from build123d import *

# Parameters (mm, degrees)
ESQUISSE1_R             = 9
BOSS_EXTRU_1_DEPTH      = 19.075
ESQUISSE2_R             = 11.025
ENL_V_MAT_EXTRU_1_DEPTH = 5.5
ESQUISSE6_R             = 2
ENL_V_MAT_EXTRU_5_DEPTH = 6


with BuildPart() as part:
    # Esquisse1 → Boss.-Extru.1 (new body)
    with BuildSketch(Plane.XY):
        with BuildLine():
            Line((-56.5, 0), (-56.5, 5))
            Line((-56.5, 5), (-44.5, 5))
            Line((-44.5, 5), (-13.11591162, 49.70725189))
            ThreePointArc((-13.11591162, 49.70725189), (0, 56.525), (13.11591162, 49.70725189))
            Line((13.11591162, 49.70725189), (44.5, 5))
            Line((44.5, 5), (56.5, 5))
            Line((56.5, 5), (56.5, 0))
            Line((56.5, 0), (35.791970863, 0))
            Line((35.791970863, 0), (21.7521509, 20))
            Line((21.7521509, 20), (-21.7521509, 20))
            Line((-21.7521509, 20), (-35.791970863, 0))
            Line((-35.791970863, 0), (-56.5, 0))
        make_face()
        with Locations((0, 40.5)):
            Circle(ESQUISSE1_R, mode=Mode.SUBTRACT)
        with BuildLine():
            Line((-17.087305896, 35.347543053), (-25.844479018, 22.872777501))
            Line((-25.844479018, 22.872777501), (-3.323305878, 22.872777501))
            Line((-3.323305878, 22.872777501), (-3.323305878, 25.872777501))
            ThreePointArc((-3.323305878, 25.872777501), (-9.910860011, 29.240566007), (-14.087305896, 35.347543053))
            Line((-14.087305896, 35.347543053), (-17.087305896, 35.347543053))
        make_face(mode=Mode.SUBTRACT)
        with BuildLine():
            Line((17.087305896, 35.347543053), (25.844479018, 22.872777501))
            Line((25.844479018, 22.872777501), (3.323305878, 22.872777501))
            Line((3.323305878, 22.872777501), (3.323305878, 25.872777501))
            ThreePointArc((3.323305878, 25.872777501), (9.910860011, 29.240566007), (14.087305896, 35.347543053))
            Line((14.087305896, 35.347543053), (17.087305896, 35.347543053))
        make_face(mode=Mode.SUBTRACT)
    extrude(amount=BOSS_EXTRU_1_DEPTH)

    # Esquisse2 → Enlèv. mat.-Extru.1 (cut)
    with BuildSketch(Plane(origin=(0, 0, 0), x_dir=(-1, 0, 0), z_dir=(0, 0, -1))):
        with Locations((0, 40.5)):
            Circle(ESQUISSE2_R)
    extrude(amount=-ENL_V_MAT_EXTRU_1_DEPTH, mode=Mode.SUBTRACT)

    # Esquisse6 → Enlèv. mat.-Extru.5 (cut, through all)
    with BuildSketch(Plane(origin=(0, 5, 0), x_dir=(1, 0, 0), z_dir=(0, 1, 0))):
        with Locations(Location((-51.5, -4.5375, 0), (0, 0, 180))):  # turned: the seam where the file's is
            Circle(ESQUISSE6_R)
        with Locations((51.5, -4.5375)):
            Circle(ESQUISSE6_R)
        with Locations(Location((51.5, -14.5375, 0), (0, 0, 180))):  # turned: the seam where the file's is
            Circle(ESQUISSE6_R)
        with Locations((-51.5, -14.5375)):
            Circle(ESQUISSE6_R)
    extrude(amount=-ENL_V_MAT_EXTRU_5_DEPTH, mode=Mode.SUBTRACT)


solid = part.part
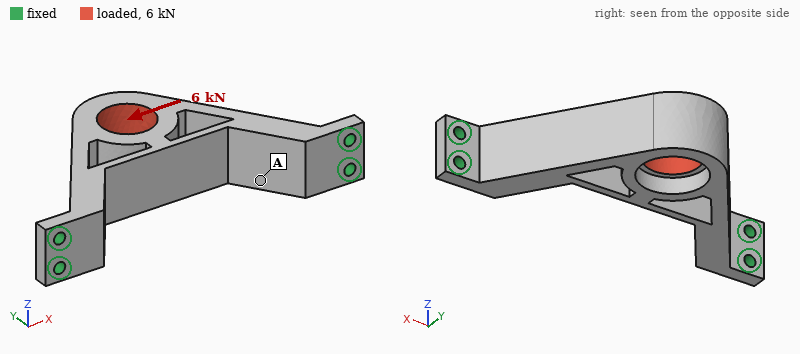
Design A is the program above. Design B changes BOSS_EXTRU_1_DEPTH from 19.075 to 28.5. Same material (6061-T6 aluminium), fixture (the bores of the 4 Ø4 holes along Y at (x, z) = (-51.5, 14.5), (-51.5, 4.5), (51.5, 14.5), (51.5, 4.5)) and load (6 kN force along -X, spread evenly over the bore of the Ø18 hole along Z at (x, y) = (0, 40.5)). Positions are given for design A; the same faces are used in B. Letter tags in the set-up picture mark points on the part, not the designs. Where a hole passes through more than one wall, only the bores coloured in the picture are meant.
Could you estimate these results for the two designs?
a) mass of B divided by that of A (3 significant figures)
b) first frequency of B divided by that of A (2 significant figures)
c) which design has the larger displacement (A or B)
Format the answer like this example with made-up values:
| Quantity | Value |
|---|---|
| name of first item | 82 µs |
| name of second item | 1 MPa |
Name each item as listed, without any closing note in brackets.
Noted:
| Quantity | Value |
|---|---|
| mass of B divided by that of A | 1.51 |
| first frequency of B divided by that of A | 0.97 |
| which design has the larger displacement | A |
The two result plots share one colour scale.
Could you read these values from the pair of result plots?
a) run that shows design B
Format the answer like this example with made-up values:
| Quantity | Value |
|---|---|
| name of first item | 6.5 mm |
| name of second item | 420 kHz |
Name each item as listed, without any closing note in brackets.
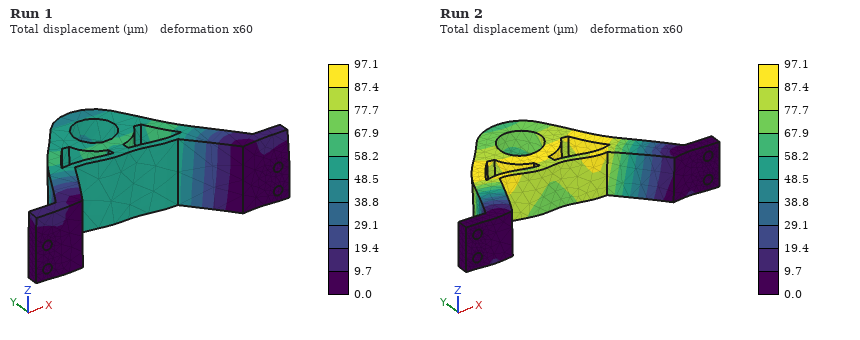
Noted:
| Quantity | Value |
|---|---|
| run that shows design B | Run 1 |
